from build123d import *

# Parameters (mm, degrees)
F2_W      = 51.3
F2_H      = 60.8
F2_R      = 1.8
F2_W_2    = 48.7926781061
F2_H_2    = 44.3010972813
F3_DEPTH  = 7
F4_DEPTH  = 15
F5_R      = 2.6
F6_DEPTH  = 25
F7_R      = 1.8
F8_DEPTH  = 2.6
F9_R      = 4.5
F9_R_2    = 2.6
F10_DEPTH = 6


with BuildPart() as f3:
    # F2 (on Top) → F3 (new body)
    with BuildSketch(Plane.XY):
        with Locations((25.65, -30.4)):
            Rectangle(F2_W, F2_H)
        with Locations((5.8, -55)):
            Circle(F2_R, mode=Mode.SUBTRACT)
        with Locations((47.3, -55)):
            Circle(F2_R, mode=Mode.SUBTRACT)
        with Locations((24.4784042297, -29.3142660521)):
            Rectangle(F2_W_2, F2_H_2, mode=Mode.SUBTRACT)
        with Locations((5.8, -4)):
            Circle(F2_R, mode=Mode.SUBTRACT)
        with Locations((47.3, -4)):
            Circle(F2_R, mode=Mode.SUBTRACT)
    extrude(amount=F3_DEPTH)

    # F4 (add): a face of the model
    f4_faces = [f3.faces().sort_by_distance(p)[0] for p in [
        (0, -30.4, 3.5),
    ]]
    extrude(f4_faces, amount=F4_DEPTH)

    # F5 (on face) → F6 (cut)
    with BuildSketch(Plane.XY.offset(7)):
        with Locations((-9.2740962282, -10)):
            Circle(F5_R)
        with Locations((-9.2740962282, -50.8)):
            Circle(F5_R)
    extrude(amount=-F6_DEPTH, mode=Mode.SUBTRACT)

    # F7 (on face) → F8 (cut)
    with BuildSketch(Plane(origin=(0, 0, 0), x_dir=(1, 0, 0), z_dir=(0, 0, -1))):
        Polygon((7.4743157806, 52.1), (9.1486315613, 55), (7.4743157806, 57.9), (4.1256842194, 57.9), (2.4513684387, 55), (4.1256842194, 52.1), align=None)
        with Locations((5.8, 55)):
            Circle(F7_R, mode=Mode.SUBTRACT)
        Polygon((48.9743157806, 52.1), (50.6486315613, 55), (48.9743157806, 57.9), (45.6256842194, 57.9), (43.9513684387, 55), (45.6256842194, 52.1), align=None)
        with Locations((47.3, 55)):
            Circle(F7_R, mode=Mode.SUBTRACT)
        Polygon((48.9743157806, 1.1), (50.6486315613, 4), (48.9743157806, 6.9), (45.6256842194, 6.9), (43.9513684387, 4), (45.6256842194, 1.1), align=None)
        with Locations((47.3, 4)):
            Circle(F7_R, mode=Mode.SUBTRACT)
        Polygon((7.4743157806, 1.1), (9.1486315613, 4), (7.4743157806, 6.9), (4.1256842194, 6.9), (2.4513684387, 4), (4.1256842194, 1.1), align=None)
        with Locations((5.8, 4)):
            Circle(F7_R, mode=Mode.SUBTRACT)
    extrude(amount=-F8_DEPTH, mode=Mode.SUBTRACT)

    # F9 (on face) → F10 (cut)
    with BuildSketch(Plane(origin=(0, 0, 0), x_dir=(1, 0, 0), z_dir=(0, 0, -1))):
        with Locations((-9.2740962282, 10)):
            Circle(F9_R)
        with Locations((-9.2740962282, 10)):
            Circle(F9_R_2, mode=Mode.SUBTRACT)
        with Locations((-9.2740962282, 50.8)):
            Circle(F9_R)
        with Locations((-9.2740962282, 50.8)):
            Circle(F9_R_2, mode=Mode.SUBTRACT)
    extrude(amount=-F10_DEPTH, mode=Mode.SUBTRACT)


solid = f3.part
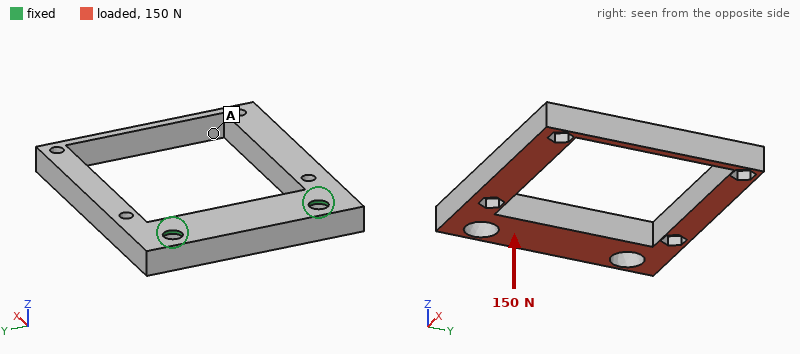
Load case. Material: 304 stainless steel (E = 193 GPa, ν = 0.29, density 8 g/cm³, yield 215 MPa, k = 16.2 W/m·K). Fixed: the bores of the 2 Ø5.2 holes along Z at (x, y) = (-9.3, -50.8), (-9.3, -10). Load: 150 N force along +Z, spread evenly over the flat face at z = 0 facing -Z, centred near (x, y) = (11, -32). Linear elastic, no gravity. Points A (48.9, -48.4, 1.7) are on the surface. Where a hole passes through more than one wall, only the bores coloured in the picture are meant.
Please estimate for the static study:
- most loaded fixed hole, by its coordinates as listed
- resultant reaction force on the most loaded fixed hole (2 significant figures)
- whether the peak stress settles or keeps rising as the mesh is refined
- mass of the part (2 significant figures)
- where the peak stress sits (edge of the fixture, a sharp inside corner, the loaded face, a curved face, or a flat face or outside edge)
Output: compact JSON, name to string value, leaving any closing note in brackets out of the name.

{"most loaded fixed hole, by its coordinates as listed": "(-9.3, -50.8)", "resultant reaction force on the most loaded fixed hole": "81 N", "whether the peak stress settles or keeps rising as the mesh is refined": "keeps rising", "mass of the part": "94 g", "where the peak stress sits": "edge of the fixture"}
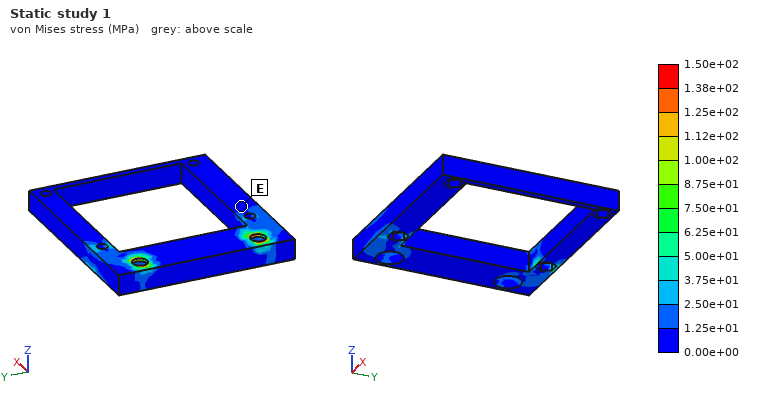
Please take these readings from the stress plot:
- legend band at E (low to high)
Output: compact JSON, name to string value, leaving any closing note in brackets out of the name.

{"legend band at E": "0.00e+00 to 1.25e+01 MPa"}
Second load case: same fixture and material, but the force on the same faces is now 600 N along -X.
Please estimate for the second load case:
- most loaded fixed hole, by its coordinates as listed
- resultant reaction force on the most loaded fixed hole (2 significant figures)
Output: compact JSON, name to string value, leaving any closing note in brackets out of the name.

{"most loaded fixed hole, by its coordinates as listed": "(-9.3, -50.8)", "resultant reaction force on the most loaded fixed hole": "320 N"}
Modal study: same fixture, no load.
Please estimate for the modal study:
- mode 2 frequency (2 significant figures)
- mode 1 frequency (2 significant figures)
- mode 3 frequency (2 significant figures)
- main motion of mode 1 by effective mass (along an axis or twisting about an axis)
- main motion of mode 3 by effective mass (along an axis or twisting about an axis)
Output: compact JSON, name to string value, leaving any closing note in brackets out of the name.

{"mode 2 frequency": "1600 Hz", "mode 1 frequency": "750 Hz", "mode 3 frequency": "1700 Hz", "main motion of mode 1 by effective mass": "along Z", "main motion of mode 3 by effective mass": "along Y"}
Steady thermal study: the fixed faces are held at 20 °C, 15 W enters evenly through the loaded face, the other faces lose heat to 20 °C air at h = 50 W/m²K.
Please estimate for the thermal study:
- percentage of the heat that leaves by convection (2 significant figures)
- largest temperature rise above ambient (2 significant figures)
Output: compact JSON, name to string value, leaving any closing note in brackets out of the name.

{"percentage of the heat that leaves by convection": "62 %", "largest temperature rise above ambient": "47 K"}
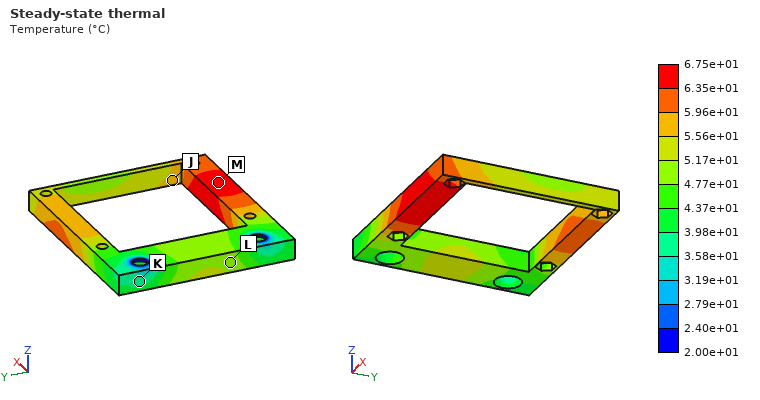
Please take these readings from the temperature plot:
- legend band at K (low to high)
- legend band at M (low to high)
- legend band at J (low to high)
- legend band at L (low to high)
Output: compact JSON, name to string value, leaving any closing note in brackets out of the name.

{"legend band at K": "3.58e+01 to 3.98e+01 °C", "legend band at M": "6.35e+01 to 6.75e+01 °C", "legend band at J": "5.56e+01 to 5.96e+01 °C", "legend band at L": "4.77e+01 to 5.17e+01 °C"}
